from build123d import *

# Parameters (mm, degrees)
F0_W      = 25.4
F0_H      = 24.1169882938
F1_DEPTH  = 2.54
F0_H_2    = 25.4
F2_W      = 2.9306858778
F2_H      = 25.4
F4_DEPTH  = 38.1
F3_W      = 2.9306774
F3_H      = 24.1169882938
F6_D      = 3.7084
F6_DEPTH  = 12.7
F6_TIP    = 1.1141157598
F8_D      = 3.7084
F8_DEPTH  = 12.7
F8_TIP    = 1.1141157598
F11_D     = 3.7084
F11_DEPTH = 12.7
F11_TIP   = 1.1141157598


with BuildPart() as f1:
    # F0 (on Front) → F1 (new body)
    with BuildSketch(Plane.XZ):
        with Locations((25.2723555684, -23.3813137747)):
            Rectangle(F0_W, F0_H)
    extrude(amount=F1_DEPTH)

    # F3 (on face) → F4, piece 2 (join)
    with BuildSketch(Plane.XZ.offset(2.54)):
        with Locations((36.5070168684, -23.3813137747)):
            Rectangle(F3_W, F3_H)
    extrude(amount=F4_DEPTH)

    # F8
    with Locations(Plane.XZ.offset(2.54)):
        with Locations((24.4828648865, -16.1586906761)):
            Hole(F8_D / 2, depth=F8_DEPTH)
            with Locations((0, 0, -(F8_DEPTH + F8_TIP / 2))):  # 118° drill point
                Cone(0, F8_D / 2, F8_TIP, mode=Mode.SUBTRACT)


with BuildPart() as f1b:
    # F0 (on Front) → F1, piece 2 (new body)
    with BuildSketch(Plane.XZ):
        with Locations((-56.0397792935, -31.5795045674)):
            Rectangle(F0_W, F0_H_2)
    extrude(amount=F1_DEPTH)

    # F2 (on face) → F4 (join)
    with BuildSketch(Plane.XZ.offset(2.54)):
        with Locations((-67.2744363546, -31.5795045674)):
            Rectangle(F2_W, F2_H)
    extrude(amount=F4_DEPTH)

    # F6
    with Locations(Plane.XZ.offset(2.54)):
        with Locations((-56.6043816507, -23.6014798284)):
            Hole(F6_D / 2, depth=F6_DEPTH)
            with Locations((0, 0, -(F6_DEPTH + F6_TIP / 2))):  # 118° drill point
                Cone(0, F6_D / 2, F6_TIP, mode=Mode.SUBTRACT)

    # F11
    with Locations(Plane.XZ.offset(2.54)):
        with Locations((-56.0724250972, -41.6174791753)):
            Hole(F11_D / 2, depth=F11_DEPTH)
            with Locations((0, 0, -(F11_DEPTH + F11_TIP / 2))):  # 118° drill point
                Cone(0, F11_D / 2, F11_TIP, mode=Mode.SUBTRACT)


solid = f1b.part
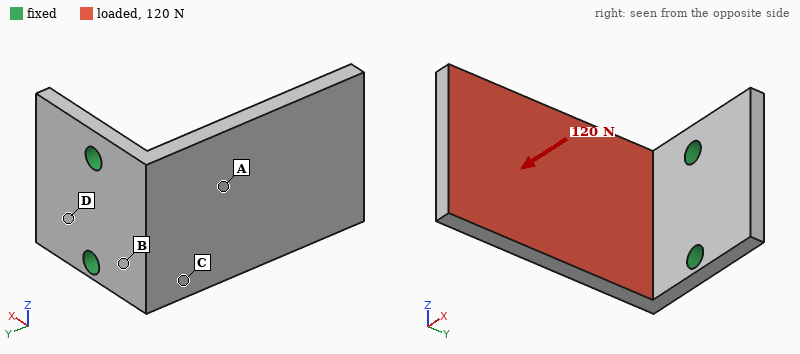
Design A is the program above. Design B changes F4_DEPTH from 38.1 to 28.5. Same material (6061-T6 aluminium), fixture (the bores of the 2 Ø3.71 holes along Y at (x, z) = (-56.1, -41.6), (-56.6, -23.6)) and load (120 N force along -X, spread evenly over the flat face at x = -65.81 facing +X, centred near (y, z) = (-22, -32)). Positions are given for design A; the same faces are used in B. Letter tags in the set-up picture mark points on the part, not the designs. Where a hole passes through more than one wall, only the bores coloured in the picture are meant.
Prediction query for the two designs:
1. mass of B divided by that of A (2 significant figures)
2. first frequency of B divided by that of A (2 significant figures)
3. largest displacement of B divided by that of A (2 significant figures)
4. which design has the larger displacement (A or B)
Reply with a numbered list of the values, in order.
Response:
1. 0.84
2. 1.6
3. 0.52
4. A
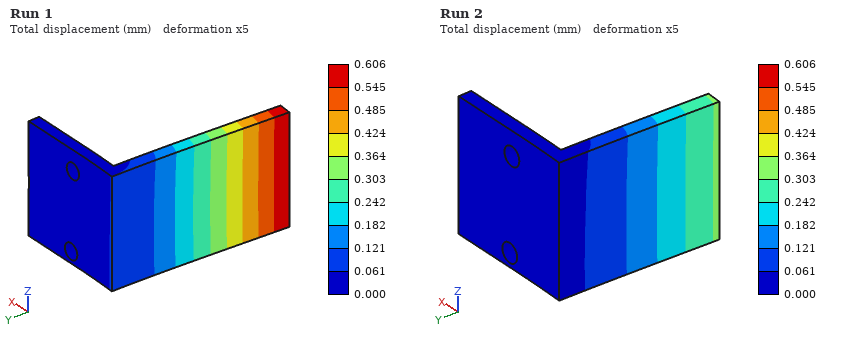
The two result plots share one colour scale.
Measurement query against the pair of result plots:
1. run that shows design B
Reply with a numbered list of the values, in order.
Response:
1. Run 2
